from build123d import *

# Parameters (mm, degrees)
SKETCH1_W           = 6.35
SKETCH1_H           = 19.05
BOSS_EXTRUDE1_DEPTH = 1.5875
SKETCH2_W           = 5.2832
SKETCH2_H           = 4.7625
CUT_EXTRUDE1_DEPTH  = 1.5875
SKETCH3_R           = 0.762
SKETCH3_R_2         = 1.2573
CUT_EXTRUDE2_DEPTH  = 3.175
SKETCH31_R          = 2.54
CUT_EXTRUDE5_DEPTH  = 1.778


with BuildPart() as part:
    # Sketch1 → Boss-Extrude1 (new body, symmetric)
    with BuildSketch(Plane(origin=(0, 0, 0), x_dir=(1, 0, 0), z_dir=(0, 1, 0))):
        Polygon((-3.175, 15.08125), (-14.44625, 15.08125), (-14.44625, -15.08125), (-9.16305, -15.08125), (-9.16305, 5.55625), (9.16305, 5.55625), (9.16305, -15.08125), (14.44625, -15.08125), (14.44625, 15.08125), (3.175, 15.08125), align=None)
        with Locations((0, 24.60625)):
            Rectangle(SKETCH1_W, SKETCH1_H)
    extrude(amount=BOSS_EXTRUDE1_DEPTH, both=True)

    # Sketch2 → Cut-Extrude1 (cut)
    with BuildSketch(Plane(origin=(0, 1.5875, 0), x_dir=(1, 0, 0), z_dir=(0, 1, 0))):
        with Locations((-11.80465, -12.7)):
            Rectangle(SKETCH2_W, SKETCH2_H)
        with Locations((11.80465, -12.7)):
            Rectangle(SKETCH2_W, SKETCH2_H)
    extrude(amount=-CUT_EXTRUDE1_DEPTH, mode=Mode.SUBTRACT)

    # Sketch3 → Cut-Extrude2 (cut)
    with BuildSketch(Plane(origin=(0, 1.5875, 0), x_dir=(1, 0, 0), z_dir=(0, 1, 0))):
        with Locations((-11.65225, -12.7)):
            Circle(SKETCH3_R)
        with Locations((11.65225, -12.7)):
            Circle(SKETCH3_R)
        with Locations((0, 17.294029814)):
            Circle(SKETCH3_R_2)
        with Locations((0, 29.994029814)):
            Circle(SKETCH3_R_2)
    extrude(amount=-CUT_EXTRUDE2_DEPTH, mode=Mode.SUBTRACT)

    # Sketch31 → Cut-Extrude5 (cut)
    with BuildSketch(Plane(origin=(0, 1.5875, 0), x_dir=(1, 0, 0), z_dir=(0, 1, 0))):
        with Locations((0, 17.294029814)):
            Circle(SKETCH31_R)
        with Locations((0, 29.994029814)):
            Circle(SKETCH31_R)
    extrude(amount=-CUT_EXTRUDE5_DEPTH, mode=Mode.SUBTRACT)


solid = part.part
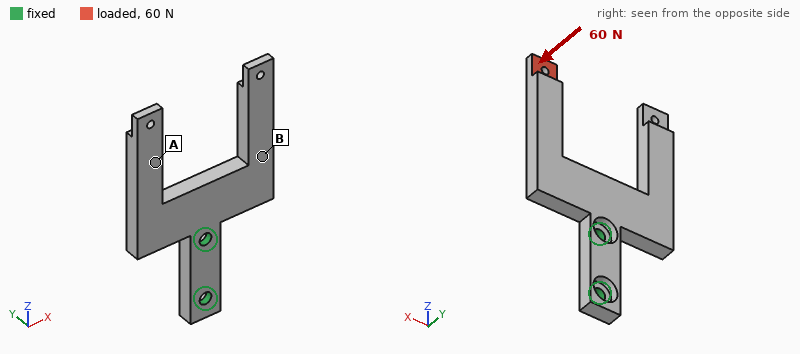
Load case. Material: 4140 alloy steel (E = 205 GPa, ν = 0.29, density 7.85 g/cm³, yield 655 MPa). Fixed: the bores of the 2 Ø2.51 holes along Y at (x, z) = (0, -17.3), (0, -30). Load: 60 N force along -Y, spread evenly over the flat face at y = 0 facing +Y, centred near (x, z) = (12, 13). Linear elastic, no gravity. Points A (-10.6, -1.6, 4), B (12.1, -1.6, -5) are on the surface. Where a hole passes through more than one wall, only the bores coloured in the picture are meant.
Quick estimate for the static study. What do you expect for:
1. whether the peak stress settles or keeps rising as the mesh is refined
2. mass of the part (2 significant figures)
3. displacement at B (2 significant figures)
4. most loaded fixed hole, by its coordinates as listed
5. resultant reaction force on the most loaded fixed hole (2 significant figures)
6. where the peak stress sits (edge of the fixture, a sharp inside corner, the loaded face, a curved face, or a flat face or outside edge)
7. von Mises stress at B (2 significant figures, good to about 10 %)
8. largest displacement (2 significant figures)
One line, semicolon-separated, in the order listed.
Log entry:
keeps rising; 14 g; 0.091 mm; (0, -17.3); 210 N; edge of the fixture; 110 MPa; 0.31 mm
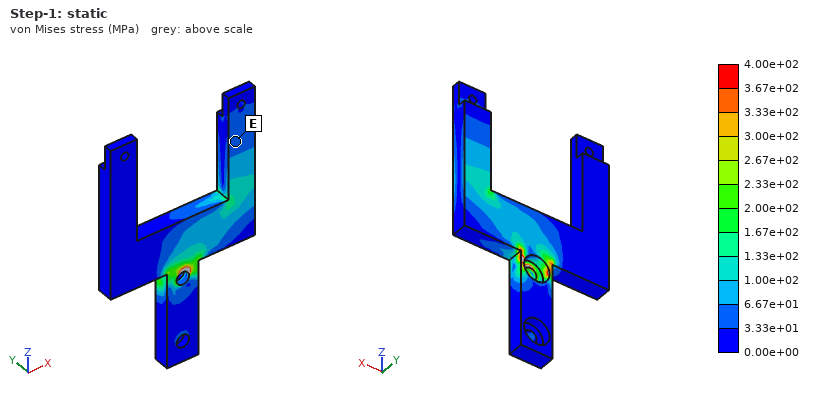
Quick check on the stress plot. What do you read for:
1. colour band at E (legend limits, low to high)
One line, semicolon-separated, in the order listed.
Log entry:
3.33e+01 to 6.67e+01 MPa
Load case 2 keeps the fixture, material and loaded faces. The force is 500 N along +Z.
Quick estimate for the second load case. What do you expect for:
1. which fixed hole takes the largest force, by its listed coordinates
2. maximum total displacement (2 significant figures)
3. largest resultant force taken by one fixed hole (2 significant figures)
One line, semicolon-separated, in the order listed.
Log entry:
(0, -17.3); 0.15 mm; 490 N
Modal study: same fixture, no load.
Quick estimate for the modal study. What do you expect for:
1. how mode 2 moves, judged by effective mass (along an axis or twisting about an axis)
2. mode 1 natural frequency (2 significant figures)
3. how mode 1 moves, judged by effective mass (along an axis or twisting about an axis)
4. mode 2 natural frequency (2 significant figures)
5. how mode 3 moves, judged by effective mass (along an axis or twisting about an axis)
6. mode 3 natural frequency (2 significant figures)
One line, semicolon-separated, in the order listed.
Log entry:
twisting about Z; 1900 Hz; along Y; 2400 Hz; along X; 3300 Hz
